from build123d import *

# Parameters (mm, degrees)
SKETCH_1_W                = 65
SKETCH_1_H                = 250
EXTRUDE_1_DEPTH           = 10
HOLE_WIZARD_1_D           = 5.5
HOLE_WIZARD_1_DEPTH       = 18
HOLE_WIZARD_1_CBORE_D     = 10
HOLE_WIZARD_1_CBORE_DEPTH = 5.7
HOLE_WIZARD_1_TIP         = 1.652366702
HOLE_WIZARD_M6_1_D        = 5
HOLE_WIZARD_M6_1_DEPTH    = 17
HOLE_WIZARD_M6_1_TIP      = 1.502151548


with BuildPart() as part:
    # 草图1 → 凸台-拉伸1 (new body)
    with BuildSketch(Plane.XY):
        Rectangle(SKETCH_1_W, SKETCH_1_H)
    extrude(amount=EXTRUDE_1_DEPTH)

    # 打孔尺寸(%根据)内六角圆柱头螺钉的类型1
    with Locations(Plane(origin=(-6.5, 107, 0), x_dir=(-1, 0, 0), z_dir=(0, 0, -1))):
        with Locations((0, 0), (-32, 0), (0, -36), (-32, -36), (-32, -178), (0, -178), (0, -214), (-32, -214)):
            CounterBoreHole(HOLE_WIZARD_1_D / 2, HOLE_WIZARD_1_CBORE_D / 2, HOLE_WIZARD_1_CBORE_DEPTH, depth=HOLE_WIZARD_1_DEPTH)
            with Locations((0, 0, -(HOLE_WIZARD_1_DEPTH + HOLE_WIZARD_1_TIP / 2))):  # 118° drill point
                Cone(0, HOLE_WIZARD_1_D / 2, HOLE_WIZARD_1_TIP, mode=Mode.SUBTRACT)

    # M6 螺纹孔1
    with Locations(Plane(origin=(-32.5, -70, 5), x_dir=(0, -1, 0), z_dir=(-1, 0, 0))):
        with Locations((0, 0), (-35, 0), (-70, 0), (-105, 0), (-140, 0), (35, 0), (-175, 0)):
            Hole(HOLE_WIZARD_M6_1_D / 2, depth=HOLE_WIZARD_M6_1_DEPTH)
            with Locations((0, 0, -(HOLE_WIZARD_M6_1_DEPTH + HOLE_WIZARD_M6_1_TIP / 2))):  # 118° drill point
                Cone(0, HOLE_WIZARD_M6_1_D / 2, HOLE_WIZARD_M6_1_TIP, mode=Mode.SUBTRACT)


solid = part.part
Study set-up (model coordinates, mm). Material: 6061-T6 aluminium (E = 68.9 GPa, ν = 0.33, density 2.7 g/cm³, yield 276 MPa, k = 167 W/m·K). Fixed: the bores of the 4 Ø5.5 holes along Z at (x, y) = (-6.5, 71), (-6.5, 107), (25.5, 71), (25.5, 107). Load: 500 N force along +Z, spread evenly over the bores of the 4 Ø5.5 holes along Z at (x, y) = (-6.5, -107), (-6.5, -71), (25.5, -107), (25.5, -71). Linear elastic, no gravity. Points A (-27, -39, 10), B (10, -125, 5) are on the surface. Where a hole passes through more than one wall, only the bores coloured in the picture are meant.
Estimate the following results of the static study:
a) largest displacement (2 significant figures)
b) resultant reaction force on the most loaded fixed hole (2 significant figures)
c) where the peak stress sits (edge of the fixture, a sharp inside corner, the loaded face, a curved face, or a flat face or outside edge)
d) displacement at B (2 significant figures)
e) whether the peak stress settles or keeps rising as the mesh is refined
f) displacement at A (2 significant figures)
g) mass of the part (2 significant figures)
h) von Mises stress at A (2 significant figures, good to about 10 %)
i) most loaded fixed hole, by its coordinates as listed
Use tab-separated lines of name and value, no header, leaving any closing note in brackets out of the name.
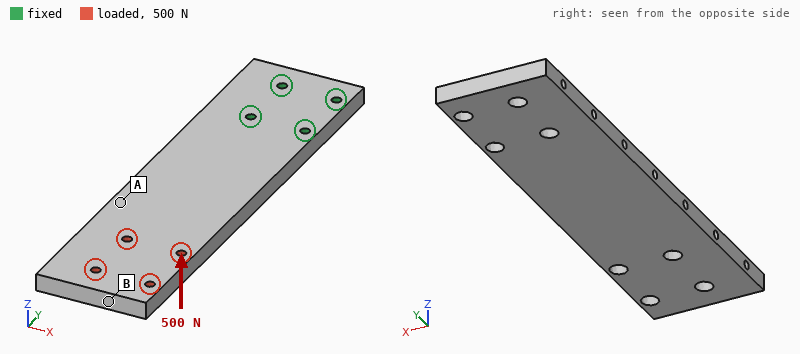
largest displacement	2.9 mm
resultant reaction force on the most loaded fixed hole	2.6 kN
where the peak stress sits	edge of the fixture
displacement at B	2.8 mm
whether the peak stress settles or keeps rising as the mesh is refined	keeps rising
displacement at A	1.2 mm
mass of the part	420 g
von Mises stress at A	23 MPa
most loaded fixed hole, by its coordinates as listed	(-6.5, 71)
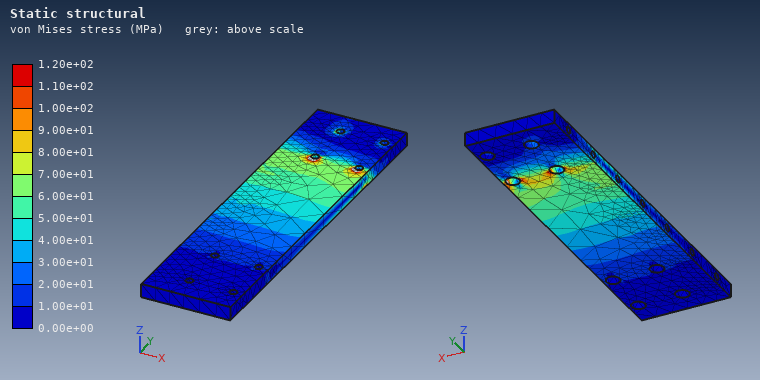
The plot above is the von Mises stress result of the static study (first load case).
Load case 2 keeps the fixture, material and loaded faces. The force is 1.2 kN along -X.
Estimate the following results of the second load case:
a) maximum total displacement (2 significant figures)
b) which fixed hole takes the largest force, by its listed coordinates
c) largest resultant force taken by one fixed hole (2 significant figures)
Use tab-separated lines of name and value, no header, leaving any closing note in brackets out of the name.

maximum total displacement	0.24 mm
which fixed hole takes the largest force, by its listed coordinates	(25.5, 71)
largest resultant force taken by one fixed hole	3.6 kN
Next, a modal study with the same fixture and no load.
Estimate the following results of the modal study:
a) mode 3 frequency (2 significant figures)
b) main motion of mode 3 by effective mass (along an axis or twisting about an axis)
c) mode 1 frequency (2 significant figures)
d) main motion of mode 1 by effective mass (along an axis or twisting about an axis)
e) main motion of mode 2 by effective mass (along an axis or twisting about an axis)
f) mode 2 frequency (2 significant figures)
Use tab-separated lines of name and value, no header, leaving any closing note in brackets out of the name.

mode 3 frequency	1200 Hz
main motion of mode 3 by effective mass	twisting about Y
mode 1 frequency	200 Hz
main motion of mode 1 by effective mass	along Z
main motion of mode 2 by effective mass	along X
mode 2 frequency	1100 Hz
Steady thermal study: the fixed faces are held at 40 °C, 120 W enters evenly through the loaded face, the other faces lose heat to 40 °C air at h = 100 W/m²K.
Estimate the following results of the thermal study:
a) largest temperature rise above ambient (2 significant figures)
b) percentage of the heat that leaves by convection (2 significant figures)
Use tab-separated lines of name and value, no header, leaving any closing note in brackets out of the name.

largest temperature rise above ambient	70 K
percentage of the heat that leaves by convection	83 %
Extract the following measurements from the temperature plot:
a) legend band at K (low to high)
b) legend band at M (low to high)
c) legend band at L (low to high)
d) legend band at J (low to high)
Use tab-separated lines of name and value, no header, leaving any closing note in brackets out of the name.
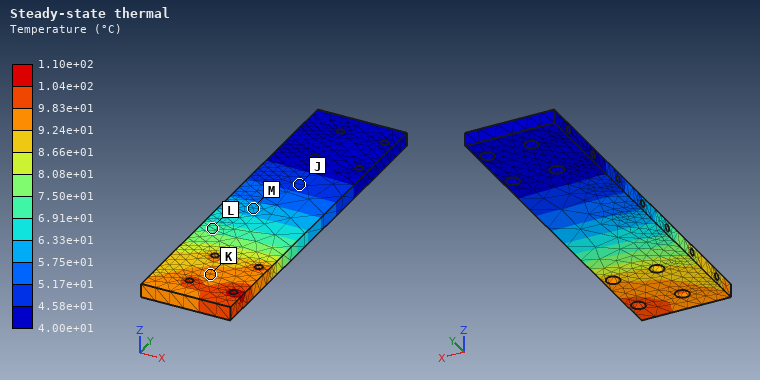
legend band at K	9.24e+01 to 9.83e+01 °C
legend band at M	5.75e+01 to 6.33e+01 °C
legend band at L	6.91e+01 to 7.50e+01 °C
legend band at J	4.58e+01 to 5.17e+01 °C
